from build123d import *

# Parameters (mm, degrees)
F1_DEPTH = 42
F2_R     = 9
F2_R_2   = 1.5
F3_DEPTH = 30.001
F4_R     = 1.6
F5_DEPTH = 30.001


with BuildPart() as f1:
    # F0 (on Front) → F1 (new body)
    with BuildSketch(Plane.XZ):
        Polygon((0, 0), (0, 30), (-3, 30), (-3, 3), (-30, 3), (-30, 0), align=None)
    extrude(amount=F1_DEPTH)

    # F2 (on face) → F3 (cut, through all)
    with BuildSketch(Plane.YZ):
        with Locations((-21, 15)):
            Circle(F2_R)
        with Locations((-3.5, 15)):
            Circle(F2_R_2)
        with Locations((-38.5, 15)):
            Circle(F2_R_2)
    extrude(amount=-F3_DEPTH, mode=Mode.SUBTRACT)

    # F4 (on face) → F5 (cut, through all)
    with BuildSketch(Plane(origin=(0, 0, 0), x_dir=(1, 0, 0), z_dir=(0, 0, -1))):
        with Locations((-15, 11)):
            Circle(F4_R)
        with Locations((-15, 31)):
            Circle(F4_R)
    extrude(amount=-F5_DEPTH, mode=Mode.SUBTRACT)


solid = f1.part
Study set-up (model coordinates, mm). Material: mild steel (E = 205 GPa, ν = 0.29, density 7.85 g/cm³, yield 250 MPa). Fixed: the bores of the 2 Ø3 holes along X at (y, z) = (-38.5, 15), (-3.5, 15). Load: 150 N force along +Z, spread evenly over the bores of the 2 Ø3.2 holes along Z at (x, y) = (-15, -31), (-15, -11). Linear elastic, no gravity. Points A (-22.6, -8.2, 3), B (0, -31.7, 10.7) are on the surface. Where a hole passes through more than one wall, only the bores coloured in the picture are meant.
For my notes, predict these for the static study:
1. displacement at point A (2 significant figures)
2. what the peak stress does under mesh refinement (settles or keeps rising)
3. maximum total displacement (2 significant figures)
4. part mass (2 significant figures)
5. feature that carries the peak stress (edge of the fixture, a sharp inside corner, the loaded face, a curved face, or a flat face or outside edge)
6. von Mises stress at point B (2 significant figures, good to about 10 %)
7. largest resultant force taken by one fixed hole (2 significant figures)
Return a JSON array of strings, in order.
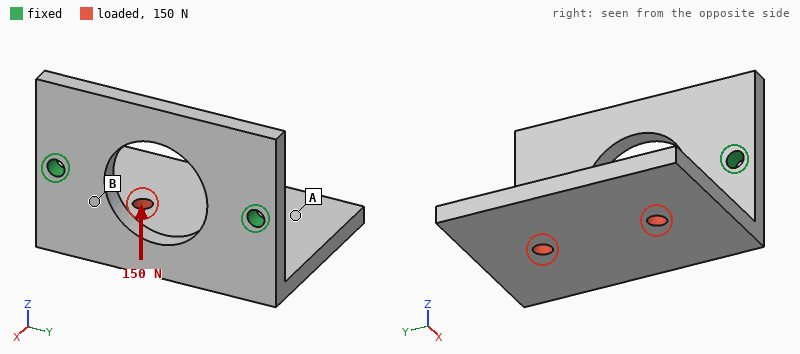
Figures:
["54 µm", "keeps rising", "75 µm", "50 g", "edge of the fixture", "45 MPa", "79 N"]
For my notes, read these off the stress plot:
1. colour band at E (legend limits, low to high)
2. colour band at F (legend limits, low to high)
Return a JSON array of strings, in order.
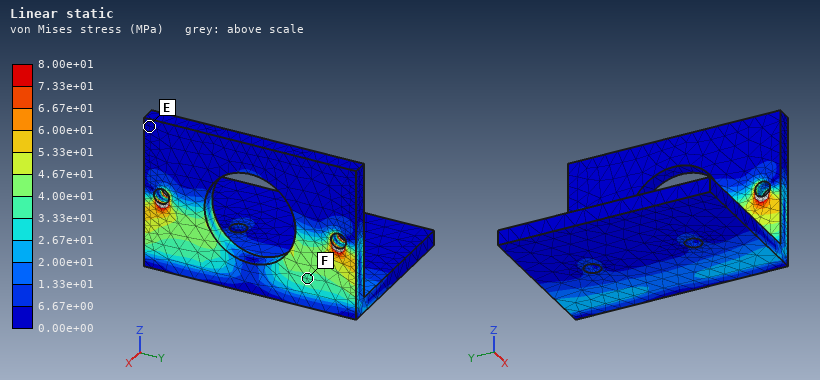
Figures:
["0.00e+00 to 6.67e+00 MPa", "3.33e+01 to 4.00e+01 MPa"]
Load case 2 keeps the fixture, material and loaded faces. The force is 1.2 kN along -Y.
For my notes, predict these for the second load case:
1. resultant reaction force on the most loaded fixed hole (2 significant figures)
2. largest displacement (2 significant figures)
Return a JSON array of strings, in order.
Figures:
["850 N", "82 µm"]
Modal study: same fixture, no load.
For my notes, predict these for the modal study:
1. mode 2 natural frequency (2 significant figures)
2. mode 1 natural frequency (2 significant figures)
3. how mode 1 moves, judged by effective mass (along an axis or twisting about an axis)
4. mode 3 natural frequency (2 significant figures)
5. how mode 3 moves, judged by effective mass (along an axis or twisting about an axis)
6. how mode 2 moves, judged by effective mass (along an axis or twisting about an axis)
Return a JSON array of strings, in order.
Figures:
["3600 Hz", "1500 Hz", "along Z", "5200 Hz", "along X", "along Y"]
